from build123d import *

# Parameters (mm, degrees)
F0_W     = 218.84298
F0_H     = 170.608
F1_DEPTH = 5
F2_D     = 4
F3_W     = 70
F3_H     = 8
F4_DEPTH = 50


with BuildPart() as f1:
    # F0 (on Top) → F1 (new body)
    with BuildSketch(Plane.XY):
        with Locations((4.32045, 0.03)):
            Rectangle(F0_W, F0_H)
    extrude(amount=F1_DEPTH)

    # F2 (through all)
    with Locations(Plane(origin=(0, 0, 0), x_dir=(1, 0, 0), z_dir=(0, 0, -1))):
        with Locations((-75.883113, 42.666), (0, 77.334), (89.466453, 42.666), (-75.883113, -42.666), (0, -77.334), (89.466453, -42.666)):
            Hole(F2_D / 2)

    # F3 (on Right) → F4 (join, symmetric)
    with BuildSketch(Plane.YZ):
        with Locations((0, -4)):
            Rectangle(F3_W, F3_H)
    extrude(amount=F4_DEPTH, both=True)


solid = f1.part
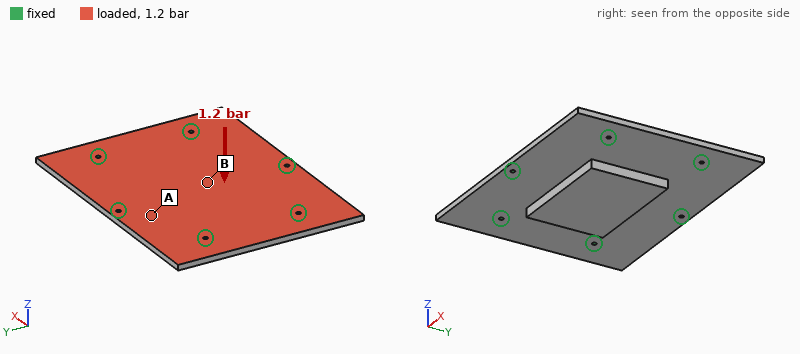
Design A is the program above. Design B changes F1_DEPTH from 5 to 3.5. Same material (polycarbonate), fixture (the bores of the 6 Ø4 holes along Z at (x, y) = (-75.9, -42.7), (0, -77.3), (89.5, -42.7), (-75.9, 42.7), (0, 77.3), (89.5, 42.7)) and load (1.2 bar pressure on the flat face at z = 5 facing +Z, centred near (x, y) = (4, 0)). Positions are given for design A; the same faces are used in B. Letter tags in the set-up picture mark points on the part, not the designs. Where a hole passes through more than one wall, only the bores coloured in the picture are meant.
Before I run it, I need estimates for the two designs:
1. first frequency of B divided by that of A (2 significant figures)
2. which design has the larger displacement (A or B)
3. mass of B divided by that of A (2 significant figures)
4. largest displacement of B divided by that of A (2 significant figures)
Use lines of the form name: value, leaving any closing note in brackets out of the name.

first frequency of B divided by that of A: 0.71
which design has the larger displacement: B
mass of B divided by that of A: 0.77
largest displacement of B divided by that of A: 2.7
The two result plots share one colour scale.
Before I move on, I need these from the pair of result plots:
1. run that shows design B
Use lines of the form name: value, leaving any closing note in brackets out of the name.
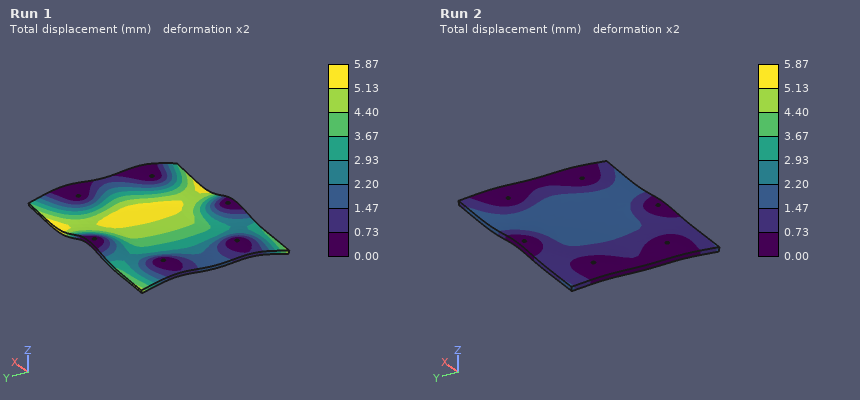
run that shows design B: Run 1
